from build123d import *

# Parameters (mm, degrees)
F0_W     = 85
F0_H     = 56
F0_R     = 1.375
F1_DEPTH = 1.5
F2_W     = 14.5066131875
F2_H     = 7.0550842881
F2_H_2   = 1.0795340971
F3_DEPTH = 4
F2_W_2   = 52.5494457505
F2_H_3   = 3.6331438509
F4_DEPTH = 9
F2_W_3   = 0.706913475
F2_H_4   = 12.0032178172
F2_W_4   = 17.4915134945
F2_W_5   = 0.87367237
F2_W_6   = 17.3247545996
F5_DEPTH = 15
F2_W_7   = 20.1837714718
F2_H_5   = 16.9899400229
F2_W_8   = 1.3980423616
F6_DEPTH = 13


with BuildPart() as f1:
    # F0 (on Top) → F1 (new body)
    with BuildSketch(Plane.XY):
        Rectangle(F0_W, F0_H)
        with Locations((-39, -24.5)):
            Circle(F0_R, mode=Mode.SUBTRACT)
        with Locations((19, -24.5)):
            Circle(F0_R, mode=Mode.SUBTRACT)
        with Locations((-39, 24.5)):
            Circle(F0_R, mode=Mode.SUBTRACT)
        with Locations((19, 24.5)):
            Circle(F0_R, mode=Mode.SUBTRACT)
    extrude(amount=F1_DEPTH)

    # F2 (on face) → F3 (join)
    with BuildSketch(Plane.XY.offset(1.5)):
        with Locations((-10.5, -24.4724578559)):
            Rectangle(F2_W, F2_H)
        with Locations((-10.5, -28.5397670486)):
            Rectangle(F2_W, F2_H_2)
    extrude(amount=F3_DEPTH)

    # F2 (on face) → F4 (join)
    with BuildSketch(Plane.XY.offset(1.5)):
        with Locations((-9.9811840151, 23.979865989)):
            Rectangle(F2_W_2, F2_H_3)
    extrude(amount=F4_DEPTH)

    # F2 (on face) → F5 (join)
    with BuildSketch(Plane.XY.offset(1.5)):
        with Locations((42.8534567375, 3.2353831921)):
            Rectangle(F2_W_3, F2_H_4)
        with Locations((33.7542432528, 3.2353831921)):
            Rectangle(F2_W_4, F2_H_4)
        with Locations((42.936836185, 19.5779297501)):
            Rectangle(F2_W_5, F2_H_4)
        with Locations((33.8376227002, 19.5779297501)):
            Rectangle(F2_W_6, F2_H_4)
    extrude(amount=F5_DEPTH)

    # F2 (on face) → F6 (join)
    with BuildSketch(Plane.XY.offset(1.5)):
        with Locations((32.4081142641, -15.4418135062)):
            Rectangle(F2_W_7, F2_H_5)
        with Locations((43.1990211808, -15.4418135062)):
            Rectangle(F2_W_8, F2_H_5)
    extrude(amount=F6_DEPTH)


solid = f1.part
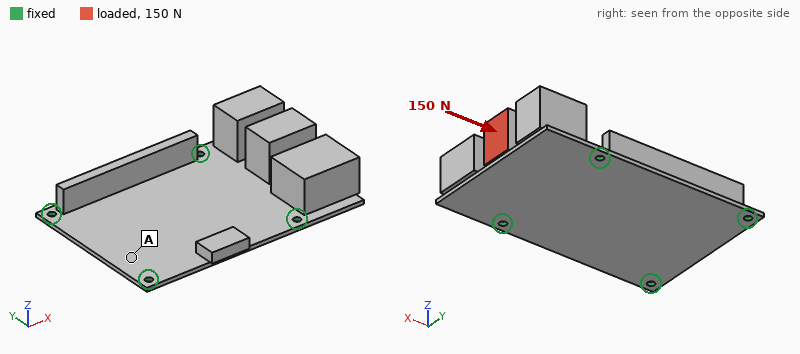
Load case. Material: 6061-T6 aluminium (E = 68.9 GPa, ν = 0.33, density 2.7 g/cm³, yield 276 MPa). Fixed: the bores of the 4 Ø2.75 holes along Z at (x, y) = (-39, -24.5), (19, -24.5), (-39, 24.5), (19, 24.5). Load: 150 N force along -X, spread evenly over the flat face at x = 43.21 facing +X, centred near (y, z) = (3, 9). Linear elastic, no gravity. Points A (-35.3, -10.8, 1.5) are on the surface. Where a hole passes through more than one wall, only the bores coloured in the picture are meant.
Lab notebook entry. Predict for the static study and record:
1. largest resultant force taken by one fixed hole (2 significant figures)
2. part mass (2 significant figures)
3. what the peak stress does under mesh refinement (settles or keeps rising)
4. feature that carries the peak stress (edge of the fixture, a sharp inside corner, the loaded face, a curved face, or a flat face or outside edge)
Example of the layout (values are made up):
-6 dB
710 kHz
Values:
56 N
56 g
keeps rising
edge of the fixture
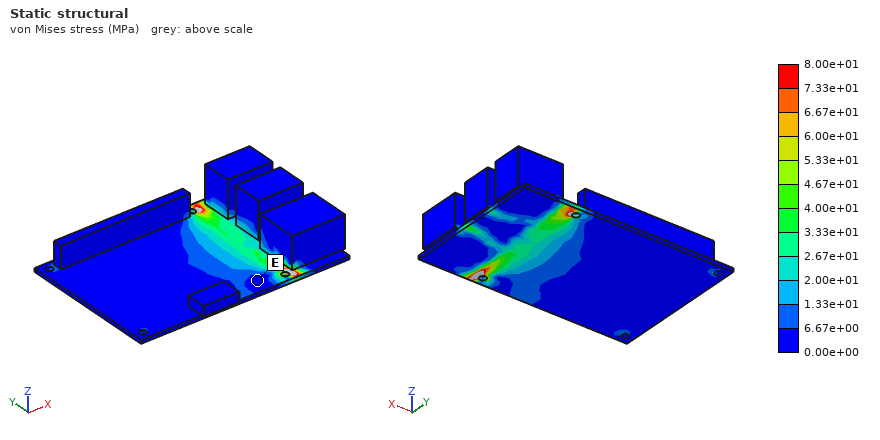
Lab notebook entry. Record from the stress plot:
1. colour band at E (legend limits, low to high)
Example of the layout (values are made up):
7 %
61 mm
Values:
0.00e+00 to 6.67e+00 MPa
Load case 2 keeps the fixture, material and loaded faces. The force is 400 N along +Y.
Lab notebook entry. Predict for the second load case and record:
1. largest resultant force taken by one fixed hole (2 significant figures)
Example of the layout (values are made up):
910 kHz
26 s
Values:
290 N
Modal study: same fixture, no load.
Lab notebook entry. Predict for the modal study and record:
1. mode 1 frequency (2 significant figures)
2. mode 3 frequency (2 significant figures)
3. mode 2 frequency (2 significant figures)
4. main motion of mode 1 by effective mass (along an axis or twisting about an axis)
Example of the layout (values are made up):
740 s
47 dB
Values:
590 Hz
2200 Hz
1700 Hz
along Z
